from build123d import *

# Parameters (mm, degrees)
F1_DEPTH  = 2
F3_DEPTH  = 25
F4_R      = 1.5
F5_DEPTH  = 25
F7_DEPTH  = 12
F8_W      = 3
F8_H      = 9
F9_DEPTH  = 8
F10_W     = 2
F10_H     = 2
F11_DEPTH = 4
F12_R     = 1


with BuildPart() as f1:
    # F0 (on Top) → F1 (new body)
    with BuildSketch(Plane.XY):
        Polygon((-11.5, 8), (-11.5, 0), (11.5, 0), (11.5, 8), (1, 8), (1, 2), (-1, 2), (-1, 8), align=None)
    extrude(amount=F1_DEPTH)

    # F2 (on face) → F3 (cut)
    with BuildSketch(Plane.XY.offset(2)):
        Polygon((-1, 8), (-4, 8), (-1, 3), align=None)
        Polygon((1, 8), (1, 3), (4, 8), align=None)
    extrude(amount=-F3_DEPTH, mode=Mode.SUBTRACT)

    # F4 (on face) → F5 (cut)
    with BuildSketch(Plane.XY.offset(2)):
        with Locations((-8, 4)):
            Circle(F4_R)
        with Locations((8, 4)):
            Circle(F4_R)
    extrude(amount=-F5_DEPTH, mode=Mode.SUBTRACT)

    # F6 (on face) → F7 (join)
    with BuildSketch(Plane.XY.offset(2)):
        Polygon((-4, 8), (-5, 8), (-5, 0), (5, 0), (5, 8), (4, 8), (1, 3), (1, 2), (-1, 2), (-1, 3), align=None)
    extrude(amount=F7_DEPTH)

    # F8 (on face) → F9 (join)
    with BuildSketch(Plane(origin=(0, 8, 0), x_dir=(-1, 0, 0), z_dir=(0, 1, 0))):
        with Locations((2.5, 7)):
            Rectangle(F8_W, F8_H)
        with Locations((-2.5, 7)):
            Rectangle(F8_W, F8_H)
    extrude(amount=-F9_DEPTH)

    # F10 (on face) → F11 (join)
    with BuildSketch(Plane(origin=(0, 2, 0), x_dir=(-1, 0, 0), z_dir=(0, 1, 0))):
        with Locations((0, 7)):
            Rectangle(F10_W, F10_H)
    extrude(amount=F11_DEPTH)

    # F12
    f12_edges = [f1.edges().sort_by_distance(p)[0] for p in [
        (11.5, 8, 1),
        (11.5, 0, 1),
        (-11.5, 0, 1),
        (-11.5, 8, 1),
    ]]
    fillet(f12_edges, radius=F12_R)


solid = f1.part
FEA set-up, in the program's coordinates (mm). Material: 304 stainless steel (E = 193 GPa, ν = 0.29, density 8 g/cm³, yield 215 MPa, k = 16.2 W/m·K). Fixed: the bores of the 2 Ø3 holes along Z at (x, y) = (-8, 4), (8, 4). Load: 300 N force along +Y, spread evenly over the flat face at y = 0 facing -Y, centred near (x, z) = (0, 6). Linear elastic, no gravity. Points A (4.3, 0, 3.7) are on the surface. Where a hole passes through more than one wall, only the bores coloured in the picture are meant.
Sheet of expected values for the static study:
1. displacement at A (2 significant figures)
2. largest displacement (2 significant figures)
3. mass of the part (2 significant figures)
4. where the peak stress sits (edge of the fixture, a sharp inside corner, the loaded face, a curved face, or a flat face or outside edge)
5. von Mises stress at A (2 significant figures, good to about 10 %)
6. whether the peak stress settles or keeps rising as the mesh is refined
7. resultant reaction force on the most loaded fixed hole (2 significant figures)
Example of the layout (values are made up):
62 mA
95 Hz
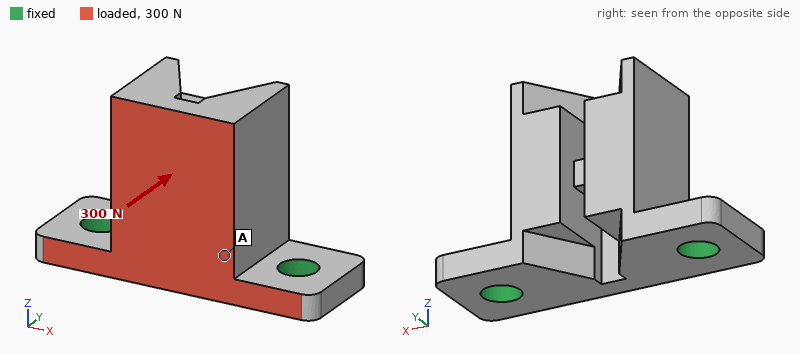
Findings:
5.6 µm
16 µm
8.6 g
edge of the fixture
22 MPa
keeps rising
160 N
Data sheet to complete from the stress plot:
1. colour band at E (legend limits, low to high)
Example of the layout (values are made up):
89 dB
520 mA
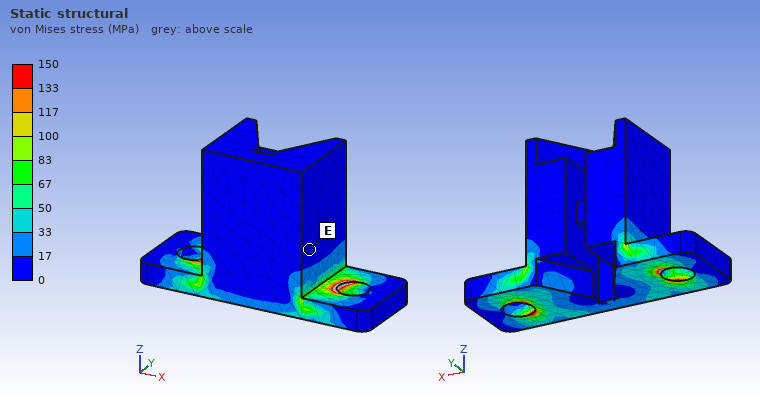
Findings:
0 to 17 MPa
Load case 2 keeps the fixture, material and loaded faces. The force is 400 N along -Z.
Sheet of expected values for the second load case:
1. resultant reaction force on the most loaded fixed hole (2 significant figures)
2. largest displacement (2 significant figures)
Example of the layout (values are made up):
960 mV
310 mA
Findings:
210 N
15 µm
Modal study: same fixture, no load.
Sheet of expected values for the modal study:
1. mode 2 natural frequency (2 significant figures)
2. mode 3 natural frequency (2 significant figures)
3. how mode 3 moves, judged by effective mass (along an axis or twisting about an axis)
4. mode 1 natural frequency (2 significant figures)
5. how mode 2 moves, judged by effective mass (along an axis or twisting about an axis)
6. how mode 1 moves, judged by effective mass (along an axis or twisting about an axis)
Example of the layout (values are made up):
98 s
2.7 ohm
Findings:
21 kHz
31 kHz
along Z
9200 Hz
along X
along Y
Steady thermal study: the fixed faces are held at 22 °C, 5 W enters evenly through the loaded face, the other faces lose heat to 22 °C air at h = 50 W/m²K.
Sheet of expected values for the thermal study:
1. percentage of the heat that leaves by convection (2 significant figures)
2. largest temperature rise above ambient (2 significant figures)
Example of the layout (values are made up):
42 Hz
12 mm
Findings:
22 %
47 K
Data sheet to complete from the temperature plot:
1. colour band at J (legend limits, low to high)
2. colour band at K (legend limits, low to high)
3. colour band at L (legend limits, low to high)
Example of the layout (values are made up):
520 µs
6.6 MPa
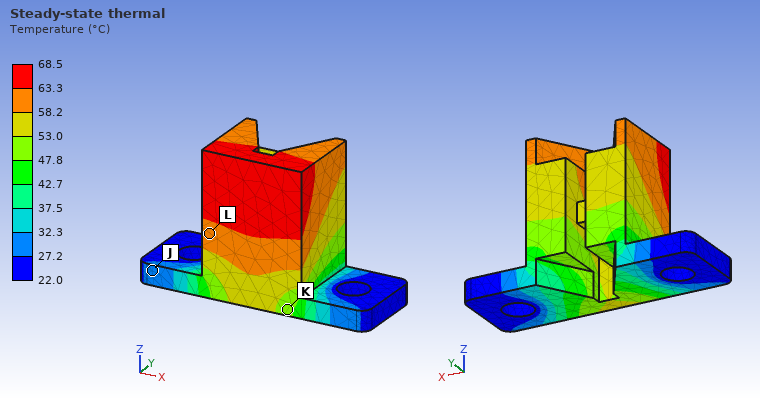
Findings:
27.2 to 32.3 °C
47.8 to 53.0 °C
58.2 to 63.3 °C
